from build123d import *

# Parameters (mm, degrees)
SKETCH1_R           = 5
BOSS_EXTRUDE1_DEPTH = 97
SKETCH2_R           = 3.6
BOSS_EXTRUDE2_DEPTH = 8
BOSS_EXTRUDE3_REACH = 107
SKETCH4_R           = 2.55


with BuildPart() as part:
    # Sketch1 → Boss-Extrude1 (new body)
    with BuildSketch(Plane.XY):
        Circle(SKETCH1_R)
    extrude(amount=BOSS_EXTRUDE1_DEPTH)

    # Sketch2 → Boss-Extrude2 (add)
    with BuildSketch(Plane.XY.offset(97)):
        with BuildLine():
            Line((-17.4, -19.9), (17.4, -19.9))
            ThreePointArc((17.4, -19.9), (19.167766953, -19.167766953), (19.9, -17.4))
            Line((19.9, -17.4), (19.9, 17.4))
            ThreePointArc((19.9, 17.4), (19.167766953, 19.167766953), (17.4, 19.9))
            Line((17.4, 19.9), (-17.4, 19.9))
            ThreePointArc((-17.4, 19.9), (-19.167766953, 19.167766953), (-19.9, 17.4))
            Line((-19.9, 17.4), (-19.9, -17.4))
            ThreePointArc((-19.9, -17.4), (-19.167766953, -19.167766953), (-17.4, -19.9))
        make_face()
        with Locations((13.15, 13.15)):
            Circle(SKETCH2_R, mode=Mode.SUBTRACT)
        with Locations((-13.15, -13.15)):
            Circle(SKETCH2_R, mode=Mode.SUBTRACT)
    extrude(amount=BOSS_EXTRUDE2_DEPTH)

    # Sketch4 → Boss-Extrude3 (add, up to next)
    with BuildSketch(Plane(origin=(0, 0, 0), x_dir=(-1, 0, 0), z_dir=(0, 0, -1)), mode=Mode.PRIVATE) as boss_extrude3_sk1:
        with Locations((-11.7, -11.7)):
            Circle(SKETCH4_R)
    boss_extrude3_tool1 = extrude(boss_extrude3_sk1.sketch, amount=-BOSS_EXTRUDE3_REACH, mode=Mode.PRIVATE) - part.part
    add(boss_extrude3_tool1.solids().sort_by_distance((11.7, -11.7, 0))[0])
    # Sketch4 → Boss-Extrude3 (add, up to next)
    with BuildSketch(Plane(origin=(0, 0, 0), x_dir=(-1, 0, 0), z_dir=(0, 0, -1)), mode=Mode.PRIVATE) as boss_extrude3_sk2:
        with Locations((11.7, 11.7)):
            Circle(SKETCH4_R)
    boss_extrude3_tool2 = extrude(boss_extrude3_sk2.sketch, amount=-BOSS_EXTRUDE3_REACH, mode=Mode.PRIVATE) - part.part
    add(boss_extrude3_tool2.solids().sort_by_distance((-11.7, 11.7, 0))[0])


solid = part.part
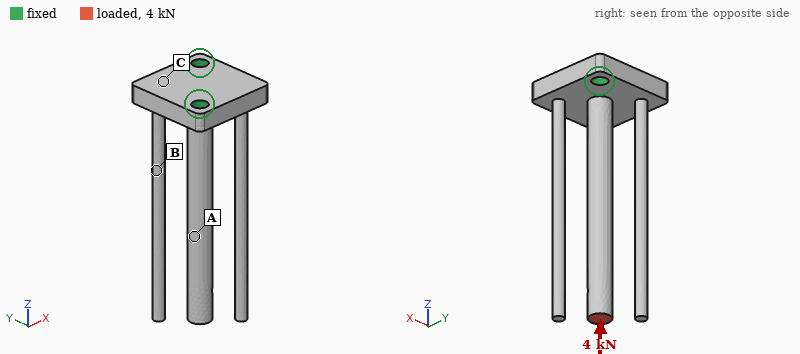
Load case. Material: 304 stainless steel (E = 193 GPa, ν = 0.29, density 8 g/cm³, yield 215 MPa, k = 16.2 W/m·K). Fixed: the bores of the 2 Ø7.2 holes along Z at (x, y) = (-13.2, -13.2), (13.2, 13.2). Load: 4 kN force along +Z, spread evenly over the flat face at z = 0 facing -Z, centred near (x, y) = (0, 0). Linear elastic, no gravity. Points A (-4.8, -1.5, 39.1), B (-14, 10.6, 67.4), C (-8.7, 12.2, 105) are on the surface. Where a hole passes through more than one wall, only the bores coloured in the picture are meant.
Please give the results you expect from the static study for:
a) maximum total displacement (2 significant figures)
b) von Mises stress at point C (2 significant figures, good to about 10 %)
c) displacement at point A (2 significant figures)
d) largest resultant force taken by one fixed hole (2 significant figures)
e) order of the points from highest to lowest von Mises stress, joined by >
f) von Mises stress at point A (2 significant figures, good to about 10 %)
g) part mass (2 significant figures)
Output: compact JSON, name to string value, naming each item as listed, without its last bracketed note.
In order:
{"maximum total displacement": "32 µm", "von Mises stress at point C": "21 MPa", "displacement at point A": "21 µm", "largest resultant force taken by one fixed hole": "2.0 kN", "order of the points from highest to lowest von Mises stress, joined by >": "A > C > B", "von Mises stress at point A": "51 MPa", "part mass": "190 g"}
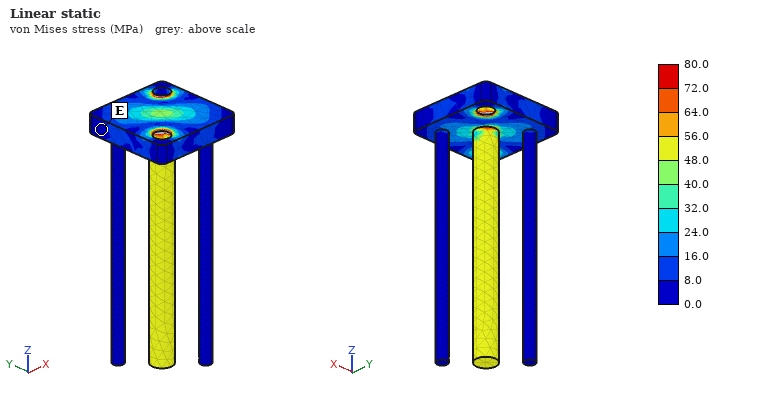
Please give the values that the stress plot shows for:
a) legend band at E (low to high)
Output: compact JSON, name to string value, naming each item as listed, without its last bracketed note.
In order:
{"legend band at E": "0.0 to 8.0 MPa"}
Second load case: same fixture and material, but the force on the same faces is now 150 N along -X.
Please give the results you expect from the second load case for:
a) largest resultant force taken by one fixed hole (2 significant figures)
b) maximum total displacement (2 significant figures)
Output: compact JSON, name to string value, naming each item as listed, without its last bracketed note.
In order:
{"largest resultant force taken by one fixed hole": "410 N", "maximum total displacement": "0.54 mm"}
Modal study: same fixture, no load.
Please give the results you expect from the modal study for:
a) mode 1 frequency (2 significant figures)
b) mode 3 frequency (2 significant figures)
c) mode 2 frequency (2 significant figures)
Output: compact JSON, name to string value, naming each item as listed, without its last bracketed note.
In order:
{"mode 1 frequency": "360 Hz", "mode 3 frequency": "360 Hz", "mode 2 frequency": "360 Hz"}
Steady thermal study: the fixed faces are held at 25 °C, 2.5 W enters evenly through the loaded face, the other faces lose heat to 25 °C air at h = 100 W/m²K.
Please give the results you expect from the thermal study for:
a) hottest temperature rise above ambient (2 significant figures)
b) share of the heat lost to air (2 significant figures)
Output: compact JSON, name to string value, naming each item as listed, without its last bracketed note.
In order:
{"hottest temperature rise above ambient": "40 K", "share of the heat lost to air": "99 %"}
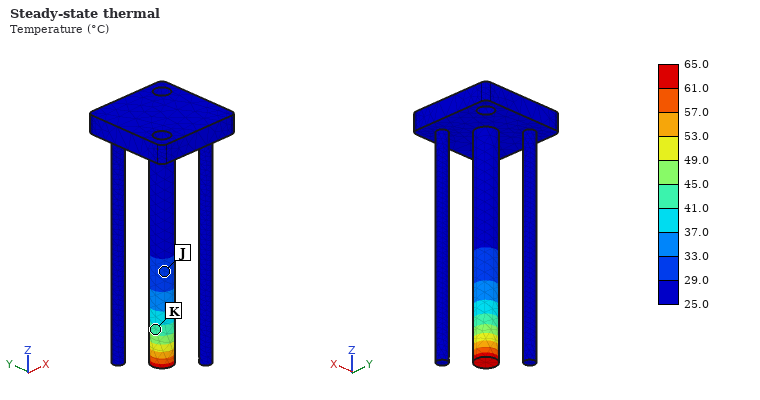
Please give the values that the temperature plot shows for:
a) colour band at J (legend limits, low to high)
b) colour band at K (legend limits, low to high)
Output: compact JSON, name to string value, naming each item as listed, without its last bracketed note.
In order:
{"colour band at J": "29.0 to 33.0 °C", "colour band at K": "41.0 to 45.0 °C"}
